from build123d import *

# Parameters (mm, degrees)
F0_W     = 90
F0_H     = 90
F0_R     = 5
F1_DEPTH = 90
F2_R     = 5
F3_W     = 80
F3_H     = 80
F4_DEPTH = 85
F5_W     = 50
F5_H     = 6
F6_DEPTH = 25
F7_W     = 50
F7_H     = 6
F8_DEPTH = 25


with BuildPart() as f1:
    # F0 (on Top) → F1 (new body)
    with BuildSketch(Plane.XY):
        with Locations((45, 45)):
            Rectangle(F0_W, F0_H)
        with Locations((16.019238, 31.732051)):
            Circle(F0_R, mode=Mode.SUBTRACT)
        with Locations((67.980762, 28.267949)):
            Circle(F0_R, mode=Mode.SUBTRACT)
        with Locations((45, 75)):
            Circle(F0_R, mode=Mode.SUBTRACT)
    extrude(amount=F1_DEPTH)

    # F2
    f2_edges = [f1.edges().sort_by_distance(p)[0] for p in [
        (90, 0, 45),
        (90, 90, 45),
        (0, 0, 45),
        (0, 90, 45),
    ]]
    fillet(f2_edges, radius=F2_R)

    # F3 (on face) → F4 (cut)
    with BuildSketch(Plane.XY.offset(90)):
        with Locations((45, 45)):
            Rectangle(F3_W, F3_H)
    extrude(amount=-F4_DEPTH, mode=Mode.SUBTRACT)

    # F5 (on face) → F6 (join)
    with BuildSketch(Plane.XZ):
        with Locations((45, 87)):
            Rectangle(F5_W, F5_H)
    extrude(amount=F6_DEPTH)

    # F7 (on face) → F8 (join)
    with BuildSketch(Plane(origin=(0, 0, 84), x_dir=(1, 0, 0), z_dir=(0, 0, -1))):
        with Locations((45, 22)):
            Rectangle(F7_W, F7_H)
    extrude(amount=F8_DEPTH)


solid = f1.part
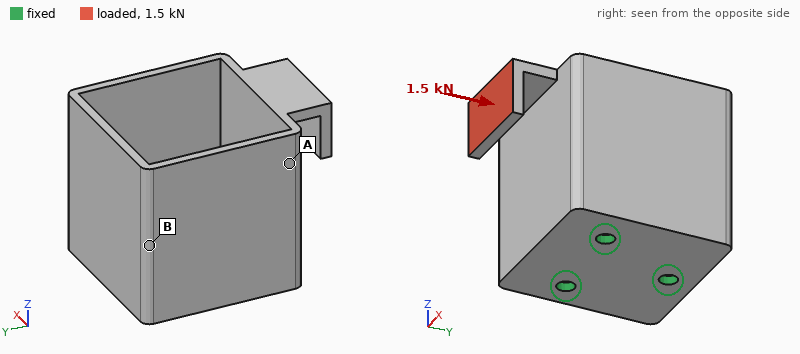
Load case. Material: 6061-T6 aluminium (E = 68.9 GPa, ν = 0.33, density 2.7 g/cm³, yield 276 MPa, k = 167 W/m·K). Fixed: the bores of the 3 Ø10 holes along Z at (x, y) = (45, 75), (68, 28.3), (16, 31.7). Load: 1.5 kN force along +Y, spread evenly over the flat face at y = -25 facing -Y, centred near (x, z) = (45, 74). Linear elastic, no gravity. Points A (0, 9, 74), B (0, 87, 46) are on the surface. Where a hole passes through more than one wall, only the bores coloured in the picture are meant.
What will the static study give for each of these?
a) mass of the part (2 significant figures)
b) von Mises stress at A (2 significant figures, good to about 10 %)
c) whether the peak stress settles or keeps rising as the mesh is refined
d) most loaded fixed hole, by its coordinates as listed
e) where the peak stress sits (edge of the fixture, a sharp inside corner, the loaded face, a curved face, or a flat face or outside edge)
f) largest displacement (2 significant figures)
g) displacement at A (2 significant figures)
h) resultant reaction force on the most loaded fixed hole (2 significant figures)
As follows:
530 g
21 MPa
keeps rising
(45, 75)
edge of the fixture
0.41 mm
0.062 mm
1.8 kN
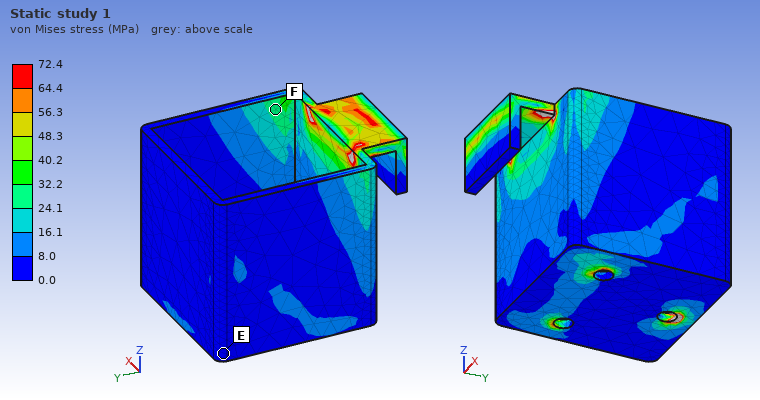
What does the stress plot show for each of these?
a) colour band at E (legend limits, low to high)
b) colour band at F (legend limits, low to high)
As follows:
0.0 to 8.0 MPa
24.1 to 32.2 MPa
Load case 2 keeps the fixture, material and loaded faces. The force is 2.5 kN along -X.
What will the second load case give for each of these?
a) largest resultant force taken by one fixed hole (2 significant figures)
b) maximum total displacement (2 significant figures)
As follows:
3.4 kN
0.44 mm
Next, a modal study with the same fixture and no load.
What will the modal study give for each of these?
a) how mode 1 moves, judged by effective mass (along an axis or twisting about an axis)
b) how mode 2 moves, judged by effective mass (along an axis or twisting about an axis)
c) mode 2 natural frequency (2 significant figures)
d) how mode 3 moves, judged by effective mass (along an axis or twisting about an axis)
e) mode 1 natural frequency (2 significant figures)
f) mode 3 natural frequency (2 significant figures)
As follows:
along X
along Y
1300 Hz
along X
1100 Hz
1400 Hz
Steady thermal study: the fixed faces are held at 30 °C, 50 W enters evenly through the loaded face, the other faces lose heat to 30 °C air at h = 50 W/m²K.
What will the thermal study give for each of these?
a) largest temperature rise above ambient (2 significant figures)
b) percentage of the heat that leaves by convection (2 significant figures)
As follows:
57 K
60 %
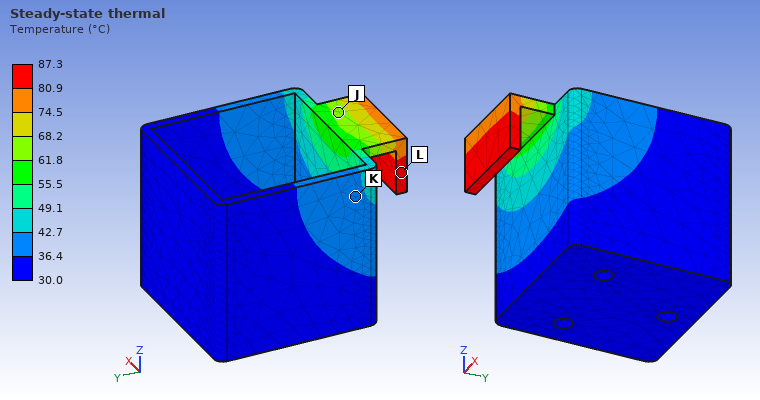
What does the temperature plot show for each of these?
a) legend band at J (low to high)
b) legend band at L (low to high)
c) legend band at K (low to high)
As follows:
61.8 to 68.2 °C
80.9 to 87.3 °C
36.4 to 42.7 °C
